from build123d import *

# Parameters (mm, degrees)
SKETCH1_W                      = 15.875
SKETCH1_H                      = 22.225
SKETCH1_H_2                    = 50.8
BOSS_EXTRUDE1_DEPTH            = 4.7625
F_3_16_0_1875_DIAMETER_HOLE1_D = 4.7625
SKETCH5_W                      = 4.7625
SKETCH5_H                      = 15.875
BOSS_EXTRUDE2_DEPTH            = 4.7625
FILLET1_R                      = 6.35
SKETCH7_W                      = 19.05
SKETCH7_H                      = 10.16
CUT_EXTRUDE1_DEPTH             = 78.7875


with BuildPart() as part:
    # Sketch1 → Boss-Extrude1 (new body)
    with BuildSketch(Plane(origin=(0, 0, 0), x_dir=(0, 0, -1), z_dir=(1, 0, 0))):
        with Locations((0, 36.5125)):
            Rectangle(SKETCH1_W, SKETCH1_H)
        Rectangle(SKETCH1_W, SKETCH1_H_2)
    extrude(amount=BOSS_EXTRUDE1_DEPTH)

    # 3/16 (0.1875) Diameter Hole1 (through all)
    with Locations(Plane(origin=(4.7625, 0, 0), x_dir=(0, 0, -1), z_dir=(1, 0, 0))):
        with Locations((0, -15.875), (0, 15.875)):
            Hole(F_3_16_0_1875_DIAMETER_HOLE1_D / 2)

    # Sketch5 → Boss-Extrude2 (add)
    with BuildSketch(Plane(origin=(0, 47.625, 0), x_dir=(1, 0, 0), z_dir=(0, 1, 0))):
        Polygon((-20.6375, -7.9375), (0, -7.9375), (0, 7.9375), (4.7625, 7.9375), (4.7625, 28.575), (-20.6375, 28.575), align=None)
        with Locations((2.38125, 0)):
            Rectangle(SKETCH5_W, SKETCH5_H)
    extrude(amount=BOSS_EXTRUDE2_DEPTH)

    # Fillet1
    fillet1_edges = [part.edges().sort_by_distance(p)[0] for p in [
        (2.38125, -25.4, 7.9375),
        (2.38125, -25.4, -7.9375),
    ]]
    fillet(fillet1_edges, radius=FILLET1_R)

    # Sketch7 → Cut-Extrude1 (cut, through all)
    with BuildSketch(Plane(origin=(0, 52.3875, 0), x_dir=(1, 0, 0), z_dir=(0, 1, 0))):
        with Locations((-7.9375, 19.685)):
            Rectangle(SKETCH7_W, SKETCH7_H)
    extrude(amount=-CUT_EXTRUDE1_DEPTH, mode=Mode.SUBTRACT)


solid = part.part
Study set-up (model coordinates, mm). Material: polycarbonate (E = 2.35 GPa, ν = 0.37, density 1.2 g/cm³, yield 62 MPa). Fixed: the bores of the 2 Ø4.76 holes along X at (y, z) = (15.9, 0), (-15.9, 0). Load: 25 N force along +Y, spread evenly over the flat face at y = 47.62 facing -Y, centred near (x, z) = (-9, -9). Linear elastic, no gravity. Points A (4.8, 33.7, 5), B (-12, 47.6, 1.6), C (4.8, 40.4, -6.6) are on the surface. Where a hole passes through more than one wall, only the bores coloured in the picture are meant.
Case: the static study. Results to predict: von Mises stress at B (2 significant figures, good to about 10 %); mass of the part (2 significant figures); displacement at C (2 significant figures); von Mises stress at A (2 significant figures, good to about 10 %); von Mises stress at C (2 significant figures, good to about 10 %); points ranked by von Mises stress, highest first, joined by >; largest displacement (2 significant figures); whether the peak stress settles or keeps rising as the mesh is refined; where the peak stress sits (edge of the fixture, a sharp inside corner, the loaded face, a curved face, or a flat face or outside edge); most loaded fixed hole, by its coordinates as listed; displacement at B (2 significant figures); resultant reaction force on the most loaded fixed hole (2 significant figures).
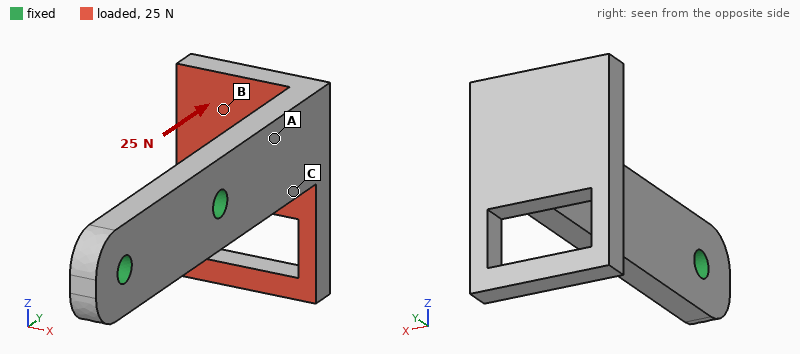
0.87 MPa
11 g
0.24 mm
5.1 MPa
3.8 MPa
A > C > B
1.1 mm
keeps rising
edge of the fixture
(15.9, 0)
0.58 mm
24 N
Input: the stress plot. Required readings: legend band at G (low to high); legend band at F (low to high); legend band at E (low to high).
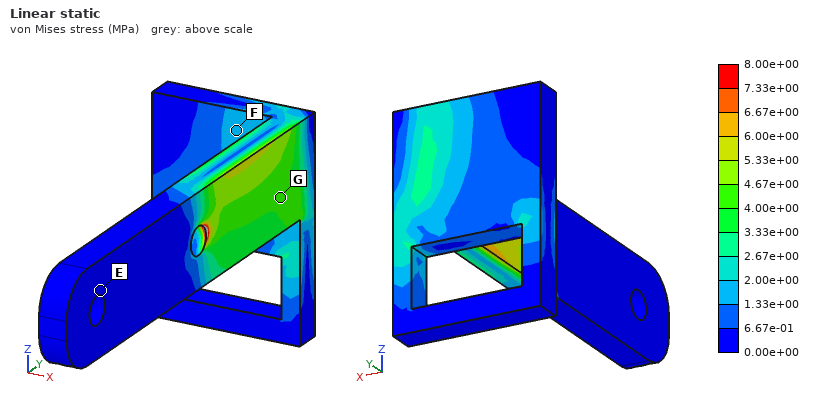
4.00e+00 to 4.67e+00 MPa
1.33e+00 to 2.00e+00 MPa
0.00e+00 to 6.67e-01 MPa
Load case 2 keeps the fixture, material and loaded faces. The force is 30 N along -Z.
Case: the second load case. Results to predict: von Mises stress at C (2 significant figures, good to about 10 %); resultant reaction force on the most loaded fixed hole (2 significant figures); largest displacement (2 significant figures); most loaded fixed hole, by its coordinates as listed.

3.3 MPa
46 N
1.1 mm
(15.9, 0)
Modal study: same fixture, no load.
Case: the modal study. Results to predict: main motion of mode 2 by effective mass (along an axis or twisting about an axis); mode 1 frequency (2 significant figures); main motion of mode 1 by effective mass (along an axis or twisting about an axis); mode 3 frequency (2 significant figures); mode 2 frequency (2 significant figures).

along Z
320 Hz
along X
960 Hz
500 Hz
